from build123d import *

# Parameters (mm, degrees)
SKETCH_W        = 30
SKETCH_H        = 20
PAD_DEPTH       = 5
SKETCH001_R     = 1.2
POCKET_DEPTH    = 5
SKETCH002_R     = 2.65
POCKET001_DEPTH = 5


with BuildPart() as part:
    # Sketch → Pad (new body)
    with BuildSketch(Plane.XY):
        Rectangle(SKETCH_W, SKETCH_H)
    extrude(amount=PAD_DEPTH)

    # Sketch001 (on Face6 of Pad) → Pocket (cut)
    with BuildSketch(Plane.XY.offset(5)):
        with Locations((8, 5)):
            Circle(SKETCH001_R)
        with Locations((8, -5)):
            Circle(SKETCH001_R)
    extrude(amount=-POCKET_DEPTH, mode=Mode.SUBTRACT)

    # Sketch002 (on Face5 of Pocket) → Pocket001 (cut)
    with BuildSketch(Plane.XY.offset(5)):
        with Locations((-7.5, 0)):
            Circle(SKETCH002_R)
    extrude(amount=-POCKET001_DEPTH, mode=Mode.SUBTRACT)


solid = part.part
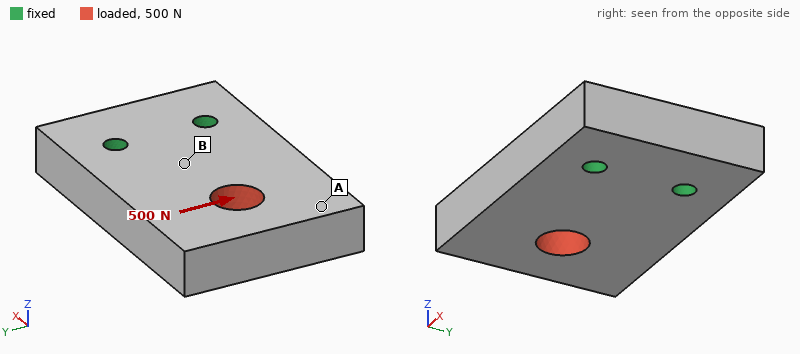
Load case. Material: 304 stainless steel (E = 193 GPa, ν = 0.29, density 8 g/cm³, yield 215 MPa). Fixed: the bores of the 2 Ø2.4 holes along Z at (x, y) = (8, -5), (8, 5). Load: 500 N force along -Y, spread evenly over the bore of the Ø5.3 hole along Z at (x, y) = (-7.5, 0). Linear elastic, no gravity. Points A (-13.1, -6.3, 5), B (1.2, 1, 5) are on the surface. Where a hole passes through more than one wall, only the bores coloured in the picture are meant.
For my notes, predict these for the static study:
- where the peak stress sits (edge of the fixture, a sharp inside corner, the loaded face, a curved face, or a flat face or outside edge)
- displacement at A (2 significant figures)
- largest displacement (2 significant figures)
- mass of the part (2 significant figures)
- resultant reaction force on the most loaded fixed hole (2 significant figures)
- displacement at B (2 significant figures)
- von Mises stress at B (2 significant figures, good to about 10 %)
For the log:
edge of the fixture
3.9 µm
4.3 µm
23 g
710 N
0.97 µm
16 MPa
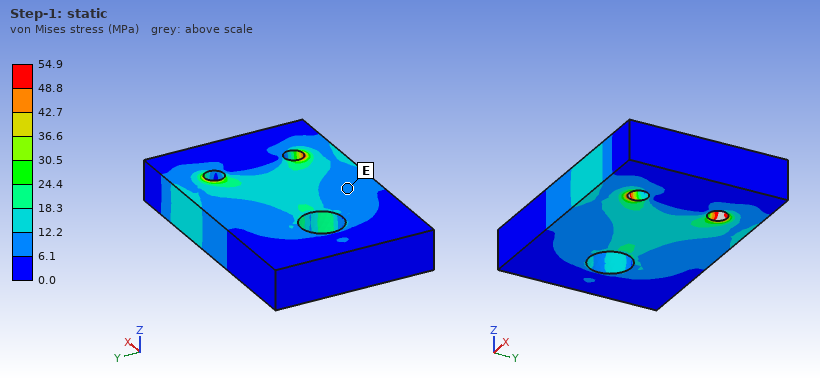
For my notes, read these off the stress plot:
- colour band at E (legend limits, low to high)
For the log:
6.1 to 12.2 MPa
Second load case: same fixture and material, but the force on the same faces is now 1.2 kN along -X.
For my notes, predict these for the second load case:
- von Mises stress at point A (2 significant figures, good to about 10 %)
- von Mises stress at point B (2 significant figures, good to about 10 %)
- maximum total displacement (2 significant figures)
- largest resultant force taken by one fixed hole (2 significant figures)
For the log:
3.4 MPa
14 MPa
1.9 µm
610 N
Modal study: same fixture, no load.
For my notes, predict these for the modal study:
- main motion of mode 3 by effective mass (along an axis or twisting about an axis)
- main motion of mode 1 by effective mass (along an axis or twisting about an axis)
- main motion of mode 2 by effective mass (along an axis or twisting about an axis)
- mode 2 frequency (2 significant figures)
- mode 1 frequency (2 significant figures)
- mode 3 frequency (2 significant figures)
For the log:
along Y
along Z
twisting about X
17 kHz
7300 Hz
18 kHz
